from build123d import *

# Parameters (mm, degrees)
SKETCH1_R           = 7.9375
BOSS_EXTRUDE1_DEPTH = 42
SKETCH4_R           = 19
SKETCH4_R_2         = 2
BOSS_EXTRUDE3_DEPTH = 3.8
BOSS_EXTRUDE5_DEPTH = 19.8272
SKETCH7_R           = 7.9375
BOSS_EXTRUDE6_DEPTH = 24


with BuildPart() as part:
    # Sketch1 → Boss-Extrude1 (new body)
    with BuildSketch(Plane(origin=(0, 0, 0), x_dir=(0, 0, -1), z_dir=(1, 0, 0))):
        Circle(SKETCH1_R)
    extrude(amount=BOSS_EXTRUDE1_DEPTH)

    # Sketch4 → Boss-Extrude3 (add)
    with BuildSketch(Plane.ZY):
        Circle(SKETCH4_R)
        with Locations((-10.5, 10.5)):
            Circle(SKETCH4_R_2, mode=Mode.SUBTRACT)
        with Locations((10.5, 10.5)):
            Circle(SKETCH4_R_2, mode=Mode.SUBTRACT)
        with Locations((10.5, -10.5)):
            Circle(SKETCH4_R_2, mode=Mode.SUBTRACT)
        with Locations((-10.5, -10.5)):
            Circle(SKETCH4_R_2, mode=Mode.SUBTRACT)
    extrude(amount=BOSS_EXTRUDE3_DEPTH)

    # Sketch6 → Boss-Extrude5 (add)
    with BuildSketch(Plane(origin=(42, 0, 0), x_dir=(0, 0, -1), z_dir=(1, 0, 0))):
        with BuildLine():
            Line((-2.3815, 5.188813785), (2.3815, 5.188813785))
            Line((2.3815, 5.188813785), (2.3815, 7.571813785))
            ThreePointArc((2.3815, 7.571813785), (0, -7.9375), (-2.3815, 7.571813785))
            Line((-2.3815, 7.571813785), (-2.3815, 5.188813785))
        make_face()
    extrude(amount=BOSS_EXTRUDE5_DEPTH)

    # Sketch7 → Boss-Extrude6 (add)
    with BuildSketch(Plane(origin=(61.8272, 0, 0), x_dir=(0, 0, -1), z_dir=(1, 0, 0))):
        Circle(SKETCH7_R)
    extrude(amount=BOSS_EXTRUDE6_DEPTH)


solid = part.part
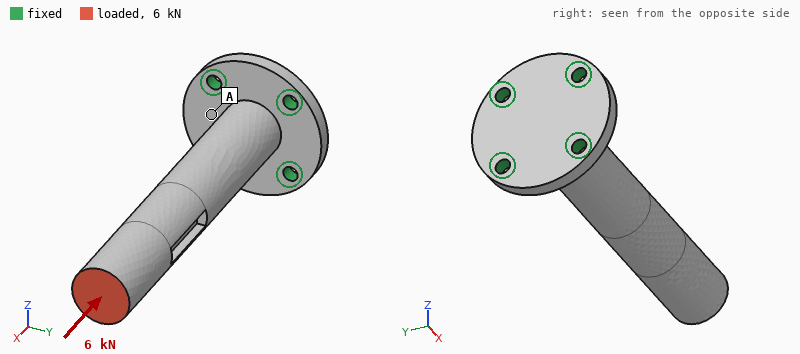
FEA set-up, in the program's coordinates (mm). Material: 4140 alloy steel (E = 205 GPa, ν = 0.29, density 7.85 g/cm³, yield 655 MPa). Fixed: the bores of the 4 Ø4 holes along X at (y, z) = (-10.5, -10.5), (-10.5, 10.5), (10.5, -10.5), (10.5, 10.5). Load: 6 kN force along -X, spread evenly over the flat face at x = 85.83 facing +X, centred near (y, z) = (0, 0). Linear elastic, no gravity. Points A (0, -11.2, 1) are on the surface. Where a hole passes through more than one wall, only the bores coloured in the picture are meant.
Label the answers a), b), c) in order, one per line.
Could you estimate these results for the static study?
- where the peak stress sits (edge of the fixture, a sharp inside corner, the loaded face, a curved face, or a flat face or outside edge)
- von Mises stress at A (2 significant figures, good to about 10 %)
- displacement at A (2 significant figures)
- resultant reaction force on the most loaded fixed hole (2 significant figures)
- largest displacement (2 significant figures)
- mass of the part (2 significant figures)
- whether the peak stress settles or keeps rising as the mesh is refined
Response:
a) edge of the fixture
b) 49 MPa
c) 5.0 µm
d) 1.6 kN
e) 23 µm
f) 160 g
g) keeps rising
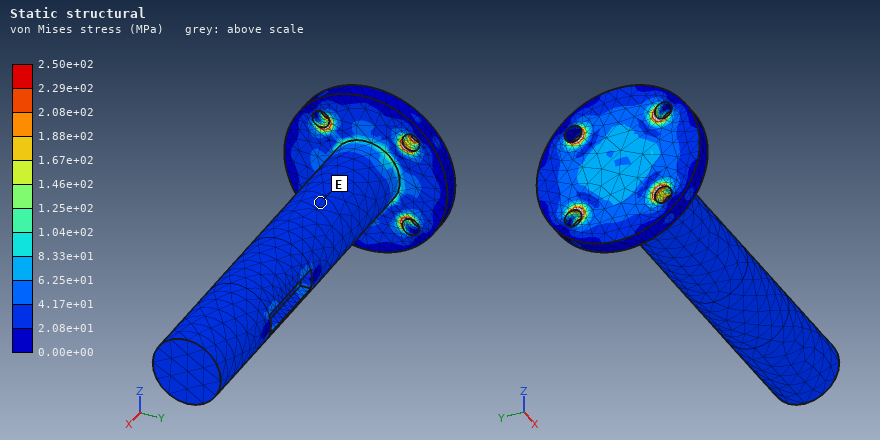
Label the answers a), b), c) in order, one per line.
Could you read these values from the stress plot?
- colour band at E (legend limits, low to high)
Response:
a) 2.08e+01 to 4.17e+01 MPa
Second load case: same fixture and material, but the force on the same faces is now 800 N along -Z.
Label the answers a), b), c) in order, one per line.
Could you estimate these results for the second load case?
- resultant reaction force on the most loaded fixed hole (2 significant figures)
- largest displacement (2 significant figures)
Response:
a) 2.0 kN
b) 0.41 mm
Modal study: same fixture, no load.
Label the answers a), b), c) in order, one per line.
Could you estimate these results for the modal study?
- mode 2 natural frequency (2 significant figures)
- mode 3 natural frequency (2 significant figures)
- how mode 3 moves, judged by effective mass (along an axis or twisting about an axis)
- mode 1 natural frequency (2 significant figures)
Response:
a) 1200 Hz
b) 7100 Hz
c) along Y
d) 1200 Hz
